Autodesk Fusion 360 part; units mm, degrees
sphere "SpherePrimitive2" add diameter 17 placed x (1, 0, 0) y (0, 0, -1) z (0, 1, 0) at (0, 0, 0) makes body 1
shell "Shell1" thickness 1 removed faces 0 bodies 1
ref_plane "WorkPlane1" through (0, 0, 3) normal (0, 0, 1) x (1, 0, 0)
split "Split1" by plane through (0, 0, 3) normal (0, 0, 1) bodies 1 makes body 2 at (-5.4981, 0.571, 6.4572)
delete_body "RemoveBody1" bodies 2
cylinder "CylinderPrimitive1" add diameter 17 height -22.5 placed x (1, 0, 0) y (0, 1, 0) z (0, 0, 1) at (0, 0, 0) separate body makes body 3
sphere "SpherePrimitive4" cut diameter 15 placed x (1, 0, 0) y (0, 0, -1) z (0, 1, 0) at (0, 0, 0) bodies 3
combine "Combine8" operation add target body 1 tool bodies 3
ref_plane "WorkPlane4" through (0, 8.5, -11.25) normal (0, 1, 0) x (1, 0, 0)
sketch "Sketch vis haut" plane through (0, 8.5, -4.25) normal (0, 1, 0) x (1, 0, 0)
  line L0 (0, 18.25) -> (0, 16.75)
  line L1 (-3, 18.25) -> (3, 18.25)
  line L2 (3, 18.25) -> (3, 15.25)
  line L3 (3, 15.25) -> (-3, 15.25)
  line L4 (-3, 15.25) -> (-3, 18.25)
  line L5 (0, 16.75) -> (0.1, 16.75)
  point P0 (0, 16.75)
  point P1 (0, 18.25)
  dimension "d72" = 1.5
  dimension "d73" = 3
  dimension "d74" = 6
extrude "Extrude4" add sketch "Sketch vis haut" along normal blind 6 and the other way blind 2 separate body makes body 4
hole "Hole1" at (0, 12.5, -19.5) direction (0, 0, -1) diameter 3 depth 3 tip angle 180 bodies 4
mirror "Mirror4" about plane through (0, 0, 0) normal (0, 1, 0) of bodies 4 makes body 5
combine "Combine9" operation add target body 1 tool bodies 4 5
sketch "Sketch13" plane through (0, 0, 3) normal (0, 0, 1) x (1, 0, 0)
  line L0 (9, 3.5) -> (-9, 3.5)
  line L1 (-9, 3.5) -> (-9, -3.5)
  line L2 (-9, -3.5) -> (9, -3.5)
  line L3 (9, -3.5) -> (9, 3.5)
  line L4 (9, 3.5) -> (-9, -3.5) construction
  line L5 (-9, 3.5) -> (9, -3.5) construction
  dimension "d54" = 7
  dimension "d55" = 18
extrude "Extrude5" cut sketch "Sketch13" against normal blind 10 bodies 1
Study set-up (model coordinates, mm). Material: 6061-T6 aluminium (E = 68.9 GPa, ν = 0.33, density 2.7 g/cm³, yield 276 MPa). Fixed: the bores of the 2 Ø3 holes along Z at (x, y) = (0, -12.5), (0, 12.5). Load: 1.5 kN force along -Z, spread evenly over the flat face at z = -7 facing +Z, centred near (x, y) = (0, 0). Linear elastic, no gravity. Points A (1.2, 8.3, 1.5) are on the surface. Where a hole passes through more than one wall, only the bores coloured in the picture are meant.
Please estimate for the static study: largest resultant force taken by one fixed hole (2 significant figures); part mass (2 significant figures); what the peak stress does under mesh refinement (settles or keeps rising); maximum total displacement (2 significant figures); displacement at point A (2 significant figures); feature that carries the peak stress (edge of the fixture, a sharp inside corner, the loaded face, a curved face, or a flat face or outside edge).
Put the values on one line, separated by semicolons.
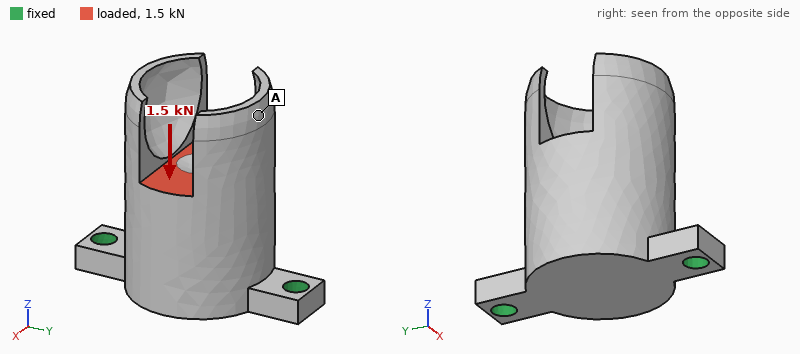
830 N; 12 g; keeps rising; 18 µm; 15 µm; edge of the fixture
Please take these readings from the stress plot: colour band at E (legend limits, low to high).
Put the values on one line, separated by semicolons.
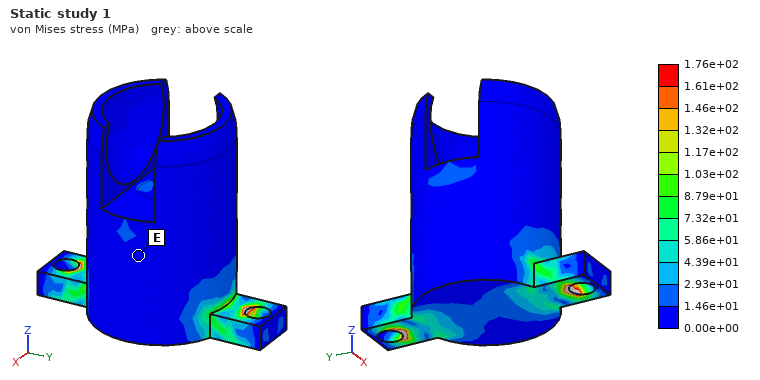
0.00e+00 to 1.46e+01 MPa
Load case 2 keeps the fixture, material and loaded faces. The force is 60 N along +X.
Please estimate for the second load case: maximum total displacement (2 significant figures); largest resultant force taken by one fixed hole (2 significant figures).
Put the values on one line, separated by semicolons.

40 µm; 30 N
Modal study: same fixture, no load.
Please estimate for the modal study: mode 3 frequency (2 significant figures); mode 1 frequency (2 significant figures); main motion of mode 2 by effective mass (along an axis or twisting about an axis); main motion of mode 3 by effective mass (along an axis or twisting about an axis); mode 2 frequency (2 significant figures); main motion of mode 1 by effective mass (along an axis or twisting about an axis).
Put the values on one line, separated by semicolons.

15 kHz; 3200 Hz; along Y; along Z; 13 kHz; along X
